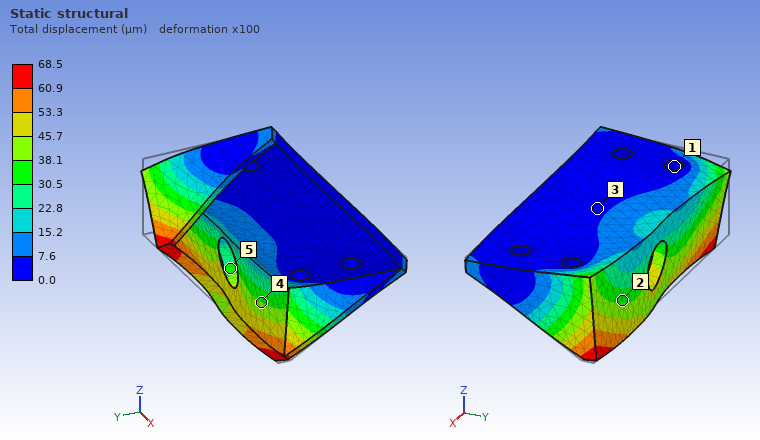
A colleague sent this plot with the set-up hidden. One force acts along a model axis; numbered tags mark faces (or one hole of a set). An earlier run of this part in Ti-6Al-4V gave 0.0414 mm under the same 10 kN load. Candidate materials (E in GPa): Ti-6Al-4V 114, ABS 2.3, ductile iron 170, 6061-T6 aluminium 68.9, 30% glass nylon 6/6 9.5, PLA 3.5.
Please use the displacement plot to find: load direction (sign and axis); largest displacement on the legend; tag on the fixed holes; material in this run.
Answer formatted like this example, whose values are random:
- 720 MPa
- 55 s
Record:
- +X
- 68.5 µm
- 1
- 6061-T6 aluminium
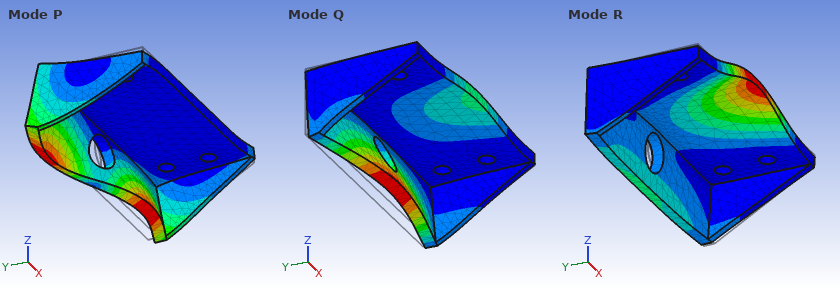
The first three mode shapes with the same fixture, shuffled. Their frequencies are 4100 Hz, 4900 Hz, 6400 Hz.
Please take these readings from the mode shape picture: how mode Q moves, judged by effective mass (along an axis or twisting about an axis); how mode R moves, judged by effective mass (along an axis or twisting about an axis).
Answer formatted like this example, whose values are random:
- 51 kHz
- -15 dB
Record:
- along Y
- along Z
